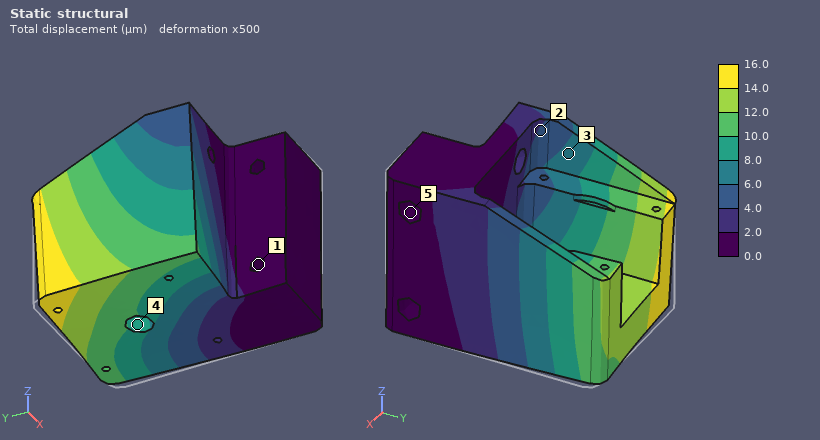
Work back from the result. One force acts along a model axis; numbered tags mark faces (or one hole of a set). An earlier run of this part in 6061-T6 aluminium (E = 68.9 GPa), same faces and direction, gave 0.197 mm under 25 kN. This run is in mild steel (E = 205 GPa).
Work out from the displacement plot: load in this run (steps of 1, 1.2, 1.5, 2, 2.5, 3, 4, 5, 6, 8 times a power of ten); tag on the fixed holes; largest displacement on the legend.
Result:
6 kN
1
16.0 µm
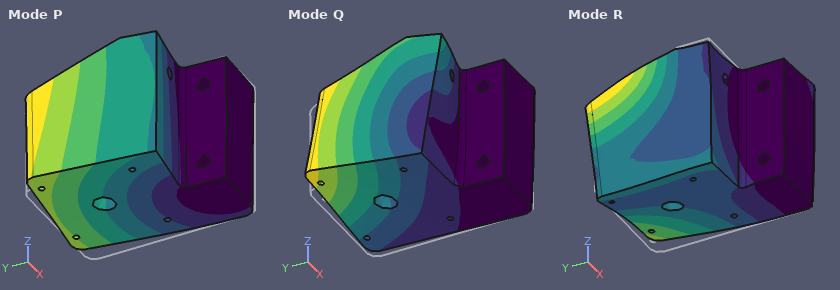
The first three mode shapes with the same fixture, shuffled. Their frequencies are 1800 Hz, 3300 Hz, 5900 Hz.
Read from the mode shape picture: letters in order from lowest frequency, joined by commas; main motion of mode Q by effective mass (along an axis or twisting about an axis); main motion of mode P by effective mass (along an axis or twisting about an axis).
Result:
P, Q, R
along Z
along X
